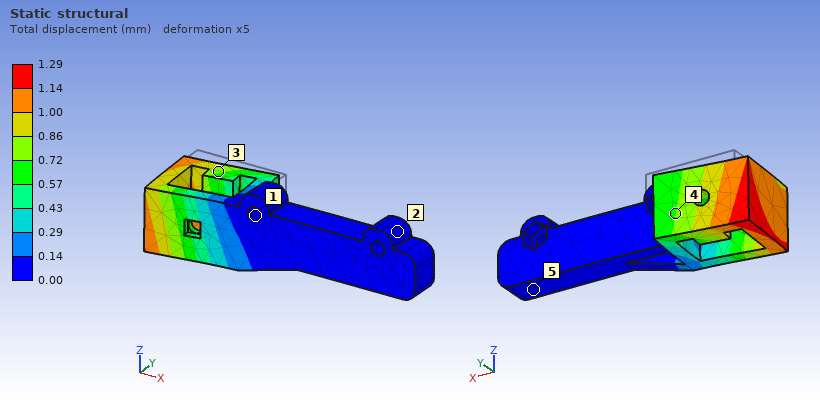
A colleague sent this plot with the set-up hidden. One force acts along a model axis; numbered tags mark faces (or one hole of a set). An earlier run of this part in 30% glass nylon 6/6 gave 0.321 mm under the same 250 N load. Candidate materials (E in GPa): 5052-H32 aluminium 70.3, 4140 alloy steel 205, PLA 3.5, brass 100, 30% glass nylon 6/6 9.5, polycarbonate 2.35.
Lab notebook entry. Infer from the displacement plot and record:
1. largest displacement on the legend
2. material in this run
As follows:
1.29 mm
polycarbonate
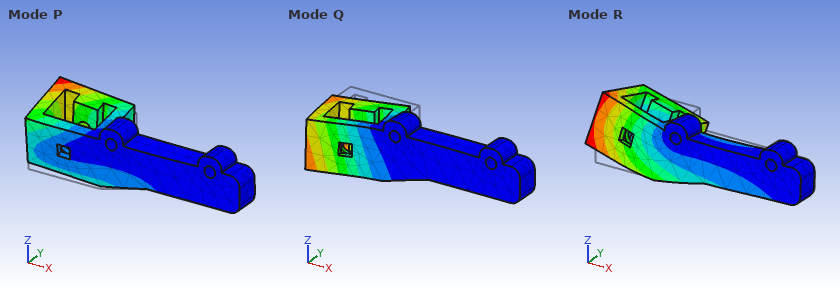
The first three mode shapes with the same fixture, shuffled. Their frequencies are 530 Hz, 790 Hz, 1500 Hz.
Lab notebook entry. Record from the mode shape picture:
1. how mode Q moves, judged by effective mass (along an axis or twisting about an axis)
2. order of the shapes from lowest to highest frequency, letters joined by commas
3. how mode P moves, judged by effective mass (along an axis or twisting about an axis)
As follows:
along Y
Q, P, R
along Z
